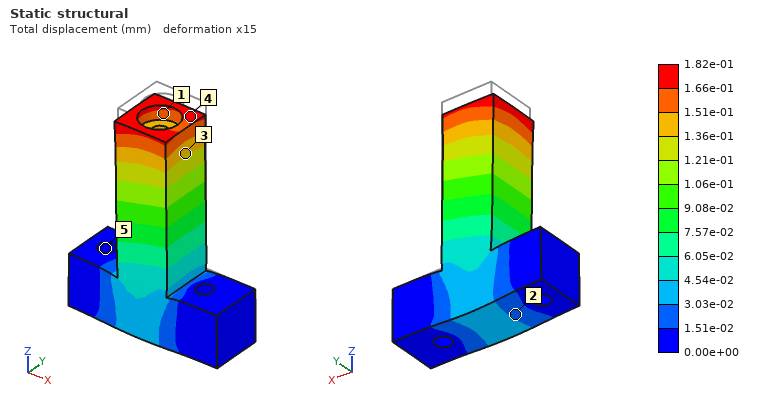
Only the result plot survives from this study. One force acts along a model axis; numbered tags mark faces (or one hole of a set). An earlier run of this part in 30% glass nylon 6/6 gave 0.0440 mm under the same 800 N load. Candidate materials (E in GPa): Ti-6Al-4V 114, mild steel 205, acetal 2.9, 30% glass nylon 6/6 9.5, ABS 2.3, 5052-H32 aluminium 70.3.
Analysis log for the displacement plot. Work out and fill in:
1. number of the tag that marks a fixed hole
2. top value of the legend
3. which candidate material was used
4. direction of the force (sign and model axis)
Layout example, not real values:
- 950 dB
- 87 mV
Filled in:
- 5
- 1.82e-01 mm
- ABS
- -Z
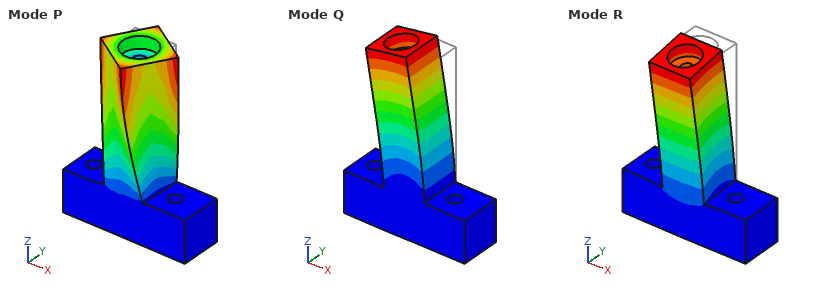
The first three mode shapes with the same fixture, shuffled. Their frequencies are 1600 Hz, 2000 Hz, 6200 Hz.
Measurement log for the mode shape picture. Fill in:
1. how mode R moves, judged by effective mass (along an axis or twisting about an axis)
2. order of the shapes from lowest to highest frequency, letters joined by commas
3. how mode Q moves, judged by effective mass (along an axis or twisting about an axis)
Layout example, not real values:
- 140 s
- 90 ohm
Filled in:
- along Y
- R, Q, P
- along X
